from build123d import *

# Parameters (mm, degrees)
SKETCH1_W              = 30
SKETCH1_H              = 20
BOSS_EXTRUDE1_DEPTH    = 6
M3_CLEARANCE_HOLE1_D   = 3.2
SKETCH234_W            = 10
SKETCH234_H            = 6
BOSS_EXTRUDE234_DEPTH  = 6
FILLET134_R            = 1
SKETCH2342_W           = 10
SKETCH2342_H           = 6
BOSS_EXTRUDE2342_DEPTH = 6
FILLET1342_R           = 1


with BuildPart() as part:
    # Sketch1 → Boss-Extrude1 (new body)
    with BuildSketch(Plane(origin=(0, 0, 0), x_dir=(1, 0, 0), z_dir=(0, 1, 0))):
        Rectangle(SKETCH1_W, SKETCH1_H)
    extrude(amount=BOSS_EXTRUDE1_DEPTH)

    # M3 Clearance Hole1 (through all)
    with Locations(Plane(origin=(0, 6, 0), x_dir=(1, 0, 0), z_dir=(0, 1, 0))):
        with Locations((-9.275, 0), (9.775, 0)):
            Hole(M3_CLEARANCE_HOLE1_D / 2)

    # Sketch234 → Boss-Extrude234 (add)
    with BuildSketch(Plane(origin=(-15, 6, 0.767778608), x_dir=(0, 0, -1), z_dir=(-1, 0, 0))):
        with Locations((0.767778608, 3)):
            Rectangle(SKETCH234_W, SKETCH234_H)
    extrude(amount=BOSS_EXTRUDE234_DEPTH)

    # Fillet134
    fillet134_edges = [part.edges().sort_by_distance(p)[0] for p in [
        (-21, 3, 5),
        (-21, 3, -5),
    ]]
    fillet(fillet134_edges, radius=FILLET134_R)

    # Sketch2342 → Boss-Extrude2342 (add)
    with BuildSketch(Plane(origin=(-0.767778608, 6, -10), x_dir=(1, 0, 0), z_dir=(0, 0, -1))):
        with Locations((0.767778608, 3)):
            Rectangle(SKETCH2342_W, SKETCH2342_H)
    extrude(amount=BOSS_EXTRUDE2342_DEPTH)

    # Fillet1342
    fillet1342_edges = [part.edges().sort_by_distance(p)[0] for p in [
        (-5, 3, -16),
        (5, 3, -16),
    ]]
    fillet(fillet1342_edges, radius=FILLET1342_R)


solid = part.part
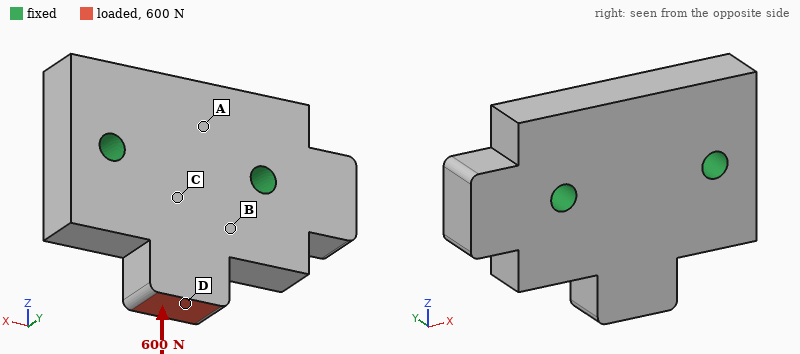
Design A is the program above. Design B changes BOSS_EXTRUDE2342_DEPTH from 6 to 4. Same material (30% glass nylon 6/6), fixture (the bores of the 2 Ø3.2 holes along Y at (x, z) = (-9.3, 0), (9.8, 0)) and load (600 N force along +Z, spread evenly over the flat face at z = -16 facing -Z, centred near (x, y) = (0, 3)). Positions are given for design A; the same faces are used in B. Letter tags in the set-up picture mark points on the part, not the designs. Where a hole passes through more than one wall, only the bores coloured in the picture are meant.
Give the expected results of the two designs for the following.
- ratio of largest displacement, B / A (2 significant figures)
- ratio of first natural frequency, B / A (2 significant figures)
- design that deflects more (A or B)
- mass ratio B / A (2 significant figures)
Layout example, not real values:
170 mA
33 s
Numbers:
0.90
1.2
A
0.97
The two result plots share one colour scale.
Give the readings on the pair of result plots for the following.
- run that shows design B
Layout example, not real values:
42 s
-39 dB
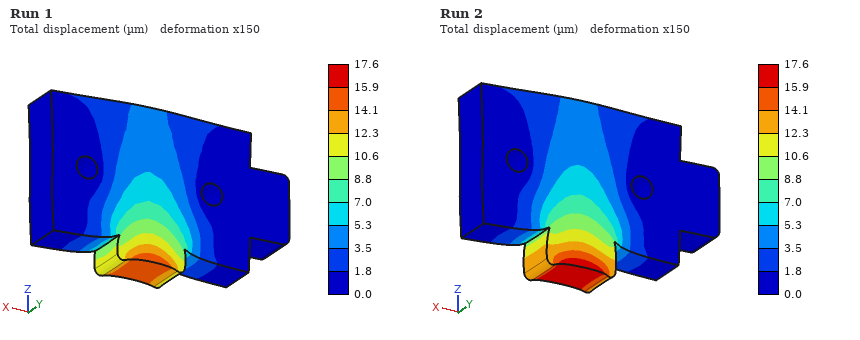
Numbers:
Run 1
